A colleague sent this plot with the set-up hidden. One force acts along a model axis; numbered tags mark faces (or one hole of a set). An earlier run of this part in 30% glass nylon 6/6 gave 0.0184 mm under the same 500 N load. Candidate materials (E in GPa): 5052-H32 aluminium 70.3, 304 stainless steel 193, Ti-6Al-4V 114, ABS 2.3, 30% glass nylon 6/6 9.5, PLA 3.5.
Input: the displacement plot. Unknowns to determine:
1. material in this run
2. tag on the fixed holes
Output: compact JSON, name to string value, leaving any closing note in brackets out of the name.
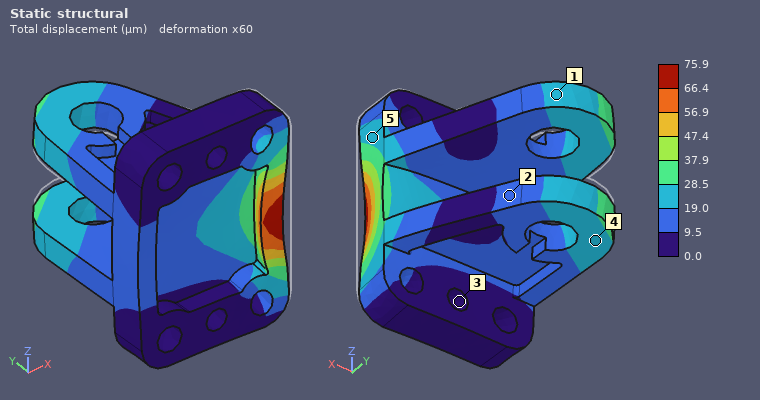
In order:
{"material in this run": "ABS", "tag on the fixed holes": "3"}
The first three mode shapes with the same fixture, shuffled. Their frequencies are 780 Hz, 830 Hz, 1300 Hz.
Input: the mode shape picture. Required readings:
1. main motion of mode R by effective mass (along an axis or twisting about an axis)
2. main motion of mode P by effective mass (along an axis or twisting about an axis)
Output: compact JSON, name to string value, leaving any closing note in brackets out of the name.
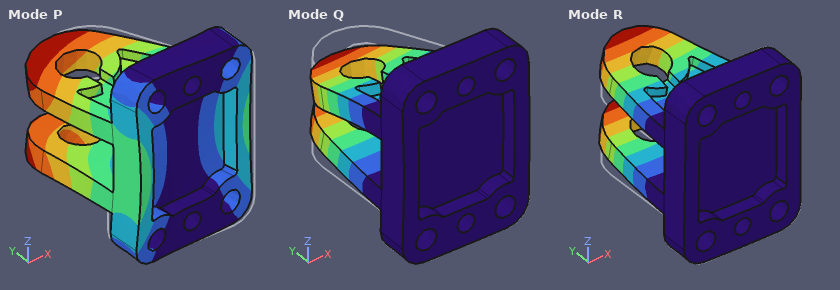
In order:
{"main motion of mode R by effective mass": "along Z", "main motion of mode P by effective mass": "along X"}
